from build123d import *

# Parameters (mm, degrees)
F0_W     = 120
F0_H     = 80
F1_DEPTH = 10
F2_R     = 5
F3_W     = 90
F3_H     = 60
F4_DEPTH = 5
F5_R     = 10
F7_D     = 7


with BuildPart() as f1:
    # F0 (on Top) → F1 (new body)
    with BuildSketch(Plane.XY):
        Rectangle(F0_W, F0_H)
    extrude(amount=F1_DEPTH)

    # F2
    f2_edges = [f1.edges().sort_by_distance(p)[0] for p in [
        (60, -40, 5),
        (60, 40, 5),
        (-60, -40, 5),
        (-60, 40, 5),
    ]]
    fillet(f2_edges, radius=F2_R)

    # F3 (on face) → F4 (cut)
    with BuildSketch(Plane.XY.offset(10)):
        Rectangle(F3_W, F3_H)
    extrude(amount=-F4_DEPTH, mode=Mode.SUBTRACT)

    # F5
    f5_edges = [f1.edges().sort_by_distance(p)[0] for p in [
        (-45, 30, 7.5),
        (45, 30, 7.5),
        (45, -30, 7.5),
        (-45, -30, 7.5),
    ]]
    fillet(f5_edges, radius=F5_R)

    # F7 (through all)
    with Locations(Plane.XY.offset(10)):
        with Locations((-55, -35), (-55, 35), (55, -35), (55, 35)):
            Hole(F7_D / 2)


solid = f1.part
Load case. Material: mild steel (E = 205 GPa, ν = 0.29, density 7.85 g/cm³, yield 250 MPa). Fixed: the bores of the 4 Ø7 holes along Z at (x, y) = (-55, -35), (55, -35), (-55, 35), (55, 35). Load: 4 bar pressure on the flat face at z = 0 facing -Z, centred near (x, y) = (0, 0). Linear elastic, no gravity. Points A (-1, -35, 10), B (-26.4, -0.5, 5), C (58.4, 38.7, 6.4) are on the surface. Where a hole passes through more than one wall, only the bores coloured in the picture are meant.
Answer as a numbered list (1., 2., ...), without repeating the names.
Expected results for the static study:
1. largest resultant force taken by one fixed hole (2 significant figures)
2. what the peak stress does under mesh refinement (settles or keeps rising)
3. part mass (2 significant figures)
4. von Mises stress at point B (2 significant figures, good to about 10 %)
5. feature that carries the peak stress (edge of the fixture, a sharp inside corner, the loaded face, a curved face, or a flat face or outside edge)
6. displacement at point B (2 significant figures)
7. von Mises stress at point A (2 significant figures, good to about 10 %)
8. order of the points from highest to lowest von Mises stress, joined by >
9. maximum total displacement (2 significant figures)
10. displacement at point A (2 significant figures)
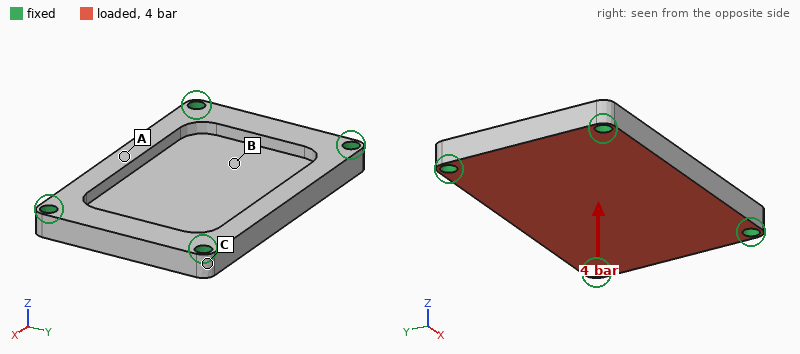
1. 1.1 kN
2. keeps rising
3. 530 g
4. 11 MPa
5. edge of the fixture
6. 20 µm
7. 29 MPa
8. A > B > C
9. 31 µm
10. 19 µm
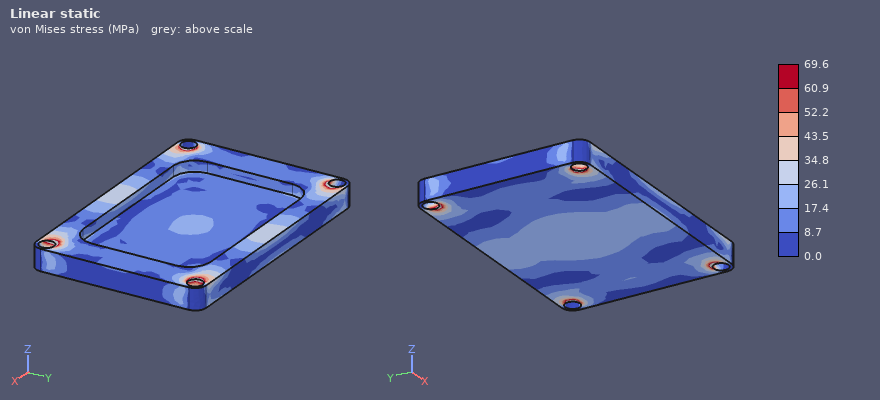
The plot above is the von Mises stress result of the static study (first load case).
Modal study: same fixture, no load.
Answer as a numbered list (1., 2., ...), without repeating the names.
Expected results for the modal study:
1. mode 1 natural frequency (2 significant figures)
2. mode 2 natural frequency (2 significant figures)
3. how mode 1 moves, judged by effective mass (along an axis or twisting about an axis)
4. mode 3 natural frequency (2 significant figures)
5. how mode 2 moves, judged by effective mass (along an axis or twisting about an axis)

1. 3400 Hz
2. 4700 Hz
3. along Z
4. 6900 Hz
5. twisting about X
